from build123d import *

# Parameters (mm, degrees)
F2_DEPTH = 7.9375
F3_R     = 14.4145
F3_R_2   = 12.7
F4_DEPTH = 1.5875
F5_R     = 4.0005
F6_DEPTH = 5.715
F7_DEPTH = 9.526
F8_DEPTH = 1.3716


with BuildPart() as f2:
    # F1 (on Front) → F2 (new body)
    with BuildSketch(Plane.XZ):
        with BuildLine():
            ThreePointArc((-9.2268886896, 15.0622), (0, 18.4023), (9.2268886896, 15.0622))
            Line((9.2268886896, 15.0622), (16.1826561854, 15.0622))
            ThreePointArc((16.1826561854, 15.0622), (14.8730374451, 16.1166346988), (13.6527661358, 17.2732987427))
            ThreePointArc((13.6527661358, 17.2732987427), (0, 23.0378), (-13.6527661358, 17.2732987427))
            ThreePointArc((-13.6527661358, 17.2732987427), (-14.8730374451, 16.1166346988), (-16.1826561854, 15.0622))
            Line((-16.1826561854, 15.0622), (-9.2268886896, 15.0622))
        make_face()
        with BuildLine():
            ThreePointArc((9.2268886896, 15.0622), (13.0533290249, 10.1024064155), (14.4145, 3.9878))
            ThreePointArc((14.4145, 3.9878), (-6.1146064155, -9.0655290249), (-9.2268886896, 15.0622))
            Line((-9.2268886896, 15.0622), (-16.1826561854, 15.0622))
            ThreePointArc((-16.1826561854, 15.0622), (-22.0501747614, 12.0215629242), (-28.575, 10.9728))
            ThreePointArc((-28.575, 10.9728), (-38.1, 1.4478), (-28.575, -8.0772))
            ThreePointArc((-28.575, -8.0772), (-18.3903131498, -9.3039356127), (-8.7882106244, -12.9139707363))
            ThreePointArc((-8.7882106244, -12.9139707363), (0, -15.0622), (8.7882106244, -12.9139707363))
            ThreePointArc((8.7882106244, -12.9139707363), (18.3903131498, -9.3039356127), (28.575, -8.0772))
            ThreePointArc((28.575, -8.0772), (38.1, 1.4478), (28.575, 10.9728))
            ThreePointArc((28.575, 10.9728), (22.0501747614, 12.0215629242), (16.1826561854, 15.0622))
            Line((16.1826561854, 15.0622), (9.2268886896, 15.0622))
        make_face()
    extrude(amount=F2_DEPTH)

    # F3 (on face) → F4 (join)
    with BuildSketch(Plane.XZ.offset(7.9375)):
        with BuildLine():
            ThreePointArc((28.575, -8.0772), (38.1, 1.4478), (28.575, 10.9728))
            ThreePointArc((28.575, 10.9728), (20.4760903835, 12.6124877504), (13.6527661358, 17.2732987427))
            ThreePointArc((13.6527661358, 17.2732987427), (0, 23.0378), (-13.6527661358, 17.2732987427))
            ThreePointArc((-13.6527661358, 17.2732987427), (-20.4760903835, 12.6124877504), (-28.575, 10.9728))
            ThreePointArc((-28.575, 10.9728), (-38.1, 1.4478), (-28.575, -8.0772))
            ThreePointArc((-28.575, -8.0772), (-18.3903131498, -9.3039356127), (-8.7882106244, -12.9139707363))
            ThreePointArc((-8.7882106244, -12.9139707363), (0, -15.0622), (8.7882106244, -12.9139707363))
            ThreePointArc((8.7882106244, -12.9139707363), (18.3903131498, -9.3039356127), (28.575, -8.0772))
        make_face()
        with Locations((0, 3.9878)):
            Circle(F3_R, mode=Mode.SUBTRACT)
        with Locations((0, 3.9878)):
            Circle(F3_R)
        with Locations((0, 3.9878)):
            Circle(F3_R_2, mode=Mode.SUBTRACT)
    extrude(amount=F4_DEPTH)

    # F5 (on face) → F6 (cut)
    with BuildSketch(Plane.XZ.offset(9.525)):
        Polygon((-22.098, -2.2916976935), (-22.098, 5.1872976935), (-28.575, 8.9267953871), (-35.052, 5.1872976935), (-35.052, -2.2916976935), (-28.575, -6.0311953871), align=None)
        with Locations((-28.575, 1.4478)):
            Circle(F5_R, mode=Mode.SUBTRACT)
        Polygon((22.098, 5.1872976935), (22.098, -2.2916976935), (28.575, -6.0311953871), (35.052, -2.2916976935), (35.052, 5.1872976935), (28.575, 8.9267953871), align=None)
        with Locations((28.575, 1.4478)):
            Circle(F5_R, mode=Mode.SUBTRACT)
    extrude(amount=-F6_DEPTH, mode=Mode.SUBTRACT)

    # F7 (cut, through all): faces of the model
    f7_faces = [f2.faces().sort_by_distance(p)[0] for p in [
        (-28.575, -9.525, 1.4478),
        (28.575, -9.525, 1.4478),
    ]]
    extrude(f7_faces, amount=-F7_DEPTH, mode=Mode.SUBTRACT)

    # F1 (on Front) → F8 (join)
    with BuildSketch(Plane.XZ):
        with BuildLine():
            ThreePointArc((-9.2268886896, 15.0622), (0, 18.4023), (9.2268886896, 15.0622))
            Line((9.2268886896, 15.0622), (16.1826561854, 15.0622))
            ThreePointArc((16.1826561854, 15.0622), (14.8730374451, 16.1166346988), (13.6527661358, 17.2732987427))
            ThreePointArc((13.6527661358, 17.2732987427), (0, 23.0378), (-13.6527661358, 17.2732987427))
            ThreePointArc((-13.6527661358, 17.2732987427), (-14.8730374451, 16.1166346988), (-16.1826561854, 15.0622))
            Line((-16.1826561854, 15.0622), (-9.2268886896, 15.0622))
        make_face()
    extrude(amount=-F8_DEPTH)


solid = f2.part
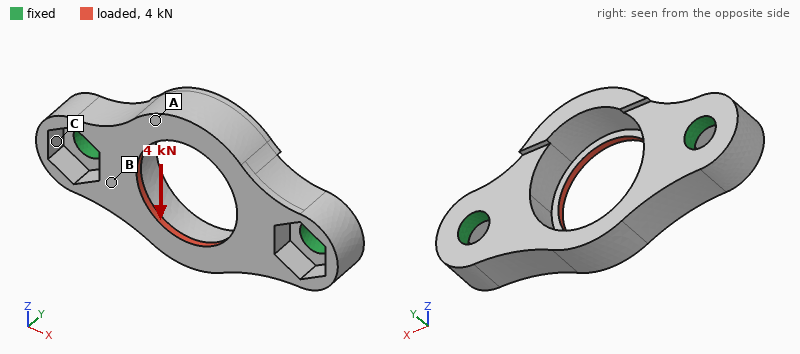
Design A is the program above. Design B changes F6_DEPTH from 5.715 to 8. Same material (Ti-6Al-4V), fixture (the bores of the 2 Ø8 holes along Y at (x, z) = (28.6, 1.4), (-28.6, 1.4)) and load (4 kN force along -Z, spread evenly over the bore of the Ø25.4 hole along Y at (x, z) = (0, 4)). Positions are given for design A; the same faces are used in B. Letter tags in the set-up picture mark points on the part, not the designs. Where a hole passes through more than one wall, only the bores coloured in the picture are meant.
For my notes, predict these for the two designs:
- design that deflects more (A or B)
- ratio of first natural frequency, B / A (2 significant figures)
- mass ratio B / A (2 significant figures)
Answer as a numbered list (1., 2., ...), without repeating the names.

1. B
2. 0.64
3. 0.96
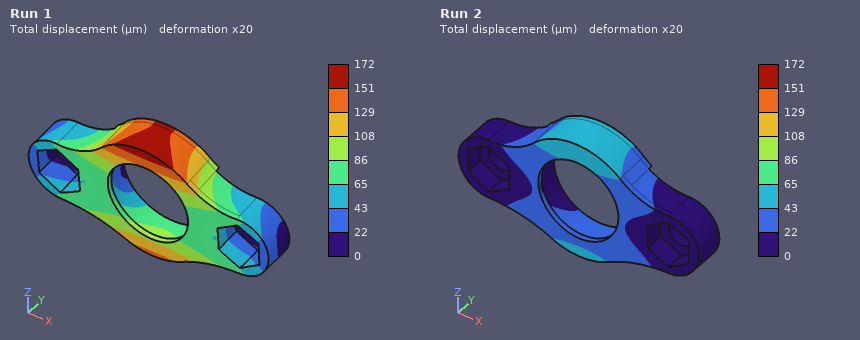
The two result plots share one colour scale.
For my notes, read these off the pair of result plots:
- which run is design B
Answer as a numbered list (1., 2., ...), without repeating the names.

1. Run 1
